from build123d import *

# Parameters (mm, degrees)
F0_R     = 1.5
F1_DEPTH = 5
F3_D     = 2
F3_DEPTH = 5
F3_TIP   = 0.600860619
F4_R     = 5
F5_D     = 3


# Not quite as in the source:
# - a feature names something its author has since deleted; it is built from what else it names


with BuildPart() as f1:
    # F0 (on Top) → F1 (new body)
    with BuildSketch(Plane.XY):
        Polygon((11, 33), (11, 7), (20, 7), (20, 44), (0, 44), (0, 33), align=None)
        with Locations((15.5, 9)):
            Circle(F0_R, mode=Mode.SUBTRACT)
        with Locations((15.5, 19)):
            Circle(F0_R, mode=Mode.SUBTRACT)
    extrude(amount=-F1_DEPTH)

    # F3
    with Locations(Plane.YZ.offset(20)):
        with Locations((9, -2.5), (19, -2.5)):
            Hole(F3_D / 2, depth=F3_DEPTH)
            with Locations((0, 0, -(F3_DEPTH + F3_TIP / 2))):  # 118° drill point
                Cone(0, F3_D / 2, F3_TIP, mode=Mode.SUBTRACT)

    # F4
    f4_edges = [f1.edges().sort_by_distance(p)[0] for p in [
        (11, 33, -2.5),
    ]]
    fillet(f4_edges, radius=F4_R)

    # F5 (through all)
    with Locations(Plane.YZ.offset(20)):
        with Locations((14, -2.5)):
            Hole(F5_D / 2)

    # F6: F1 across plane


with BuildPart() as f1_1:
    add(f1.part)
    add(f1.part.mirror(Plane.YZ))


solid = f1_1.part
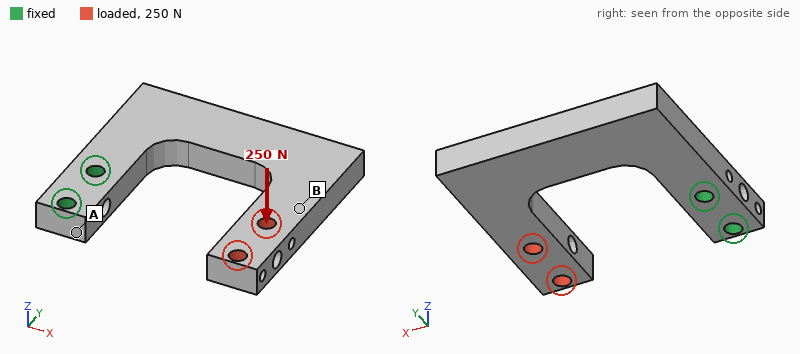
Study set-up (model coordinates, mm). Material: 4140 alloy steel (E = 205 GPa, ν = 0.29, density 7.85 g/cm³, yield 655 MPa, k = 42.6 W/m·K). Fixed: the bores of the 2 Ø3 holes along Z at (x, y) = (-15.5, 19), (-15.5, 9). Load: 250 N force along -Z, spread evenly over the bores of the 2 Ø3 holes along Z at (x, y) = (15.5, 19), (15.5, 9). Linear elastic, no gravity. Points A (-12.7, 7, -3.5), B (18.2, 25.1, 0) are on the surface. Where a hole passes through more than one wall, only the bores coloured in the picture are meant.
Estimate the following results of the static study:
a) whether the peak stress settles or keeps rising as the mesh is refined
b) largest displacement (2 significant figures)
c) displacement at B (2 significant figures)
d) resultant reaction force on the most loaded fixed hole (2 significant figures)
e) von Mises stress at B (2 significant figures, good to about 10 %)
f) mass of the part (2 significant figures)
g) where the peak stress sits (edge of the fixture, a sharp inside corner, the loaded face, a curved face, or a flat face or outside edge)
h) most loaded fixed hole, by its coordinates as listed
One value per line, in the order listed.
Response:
keeps rising
0.59 mm
0.37 mm
240 N
72 MPa
34 g
edge of the fixture
(-15.5, 19)
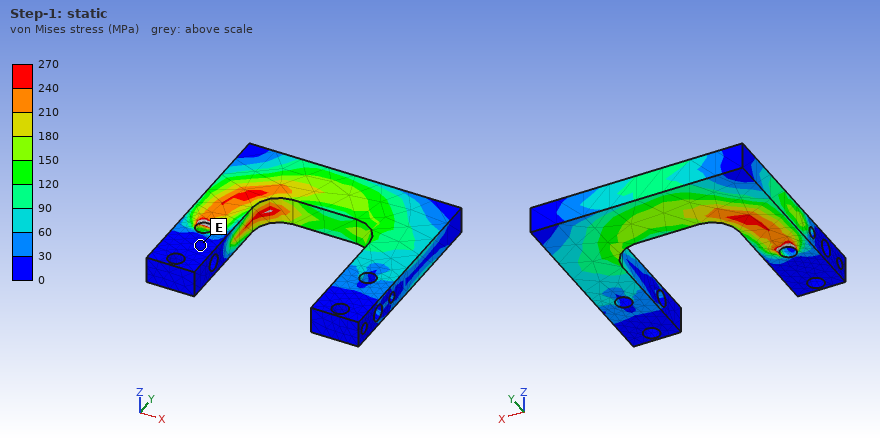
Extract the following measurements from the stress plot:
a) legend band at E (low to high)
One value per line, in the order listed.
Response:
0 to 30 MPa
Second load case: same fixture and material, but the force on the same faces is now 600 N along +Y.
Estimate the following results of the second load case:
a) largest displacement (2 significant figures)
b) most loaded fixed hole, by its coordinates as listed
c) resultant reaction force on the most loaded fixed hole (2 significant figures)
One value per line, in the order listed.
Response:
0.29 mm
(-15.5, 19)
900 N
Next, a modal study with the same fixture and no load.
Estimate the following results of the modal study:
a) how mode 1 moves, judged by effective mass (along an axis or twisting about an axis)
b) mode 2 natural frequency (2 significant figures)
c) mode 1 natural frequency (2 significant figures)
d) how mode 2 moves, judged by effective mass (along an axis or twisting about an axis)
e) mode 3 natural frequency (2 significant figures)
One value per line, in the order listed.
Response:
along Z
2000 Hz
1200 Hz
along Y
2500 Hz
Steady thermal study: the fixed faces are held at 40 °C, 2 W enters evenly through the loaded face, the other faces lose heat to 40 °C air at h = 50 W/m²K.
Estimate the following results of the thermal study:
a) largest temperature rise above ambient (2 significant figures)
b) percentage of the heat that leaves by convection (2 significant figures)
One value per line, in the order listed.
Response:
29 K
75 %
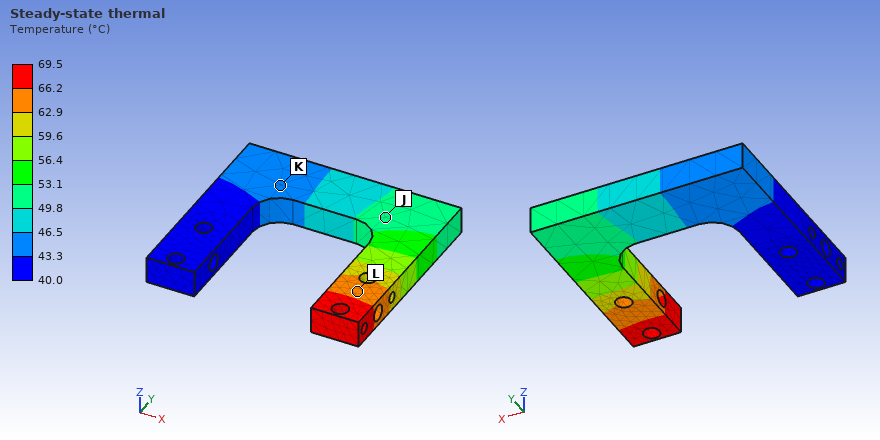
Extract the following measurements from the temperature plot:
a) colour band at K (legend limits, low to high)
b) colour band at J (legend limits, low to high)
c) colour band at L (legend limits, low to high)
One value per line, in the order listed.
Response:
43.3 to 46.5 °C
49.8 to 53.1 °C
62.9 to 66.2 °C
